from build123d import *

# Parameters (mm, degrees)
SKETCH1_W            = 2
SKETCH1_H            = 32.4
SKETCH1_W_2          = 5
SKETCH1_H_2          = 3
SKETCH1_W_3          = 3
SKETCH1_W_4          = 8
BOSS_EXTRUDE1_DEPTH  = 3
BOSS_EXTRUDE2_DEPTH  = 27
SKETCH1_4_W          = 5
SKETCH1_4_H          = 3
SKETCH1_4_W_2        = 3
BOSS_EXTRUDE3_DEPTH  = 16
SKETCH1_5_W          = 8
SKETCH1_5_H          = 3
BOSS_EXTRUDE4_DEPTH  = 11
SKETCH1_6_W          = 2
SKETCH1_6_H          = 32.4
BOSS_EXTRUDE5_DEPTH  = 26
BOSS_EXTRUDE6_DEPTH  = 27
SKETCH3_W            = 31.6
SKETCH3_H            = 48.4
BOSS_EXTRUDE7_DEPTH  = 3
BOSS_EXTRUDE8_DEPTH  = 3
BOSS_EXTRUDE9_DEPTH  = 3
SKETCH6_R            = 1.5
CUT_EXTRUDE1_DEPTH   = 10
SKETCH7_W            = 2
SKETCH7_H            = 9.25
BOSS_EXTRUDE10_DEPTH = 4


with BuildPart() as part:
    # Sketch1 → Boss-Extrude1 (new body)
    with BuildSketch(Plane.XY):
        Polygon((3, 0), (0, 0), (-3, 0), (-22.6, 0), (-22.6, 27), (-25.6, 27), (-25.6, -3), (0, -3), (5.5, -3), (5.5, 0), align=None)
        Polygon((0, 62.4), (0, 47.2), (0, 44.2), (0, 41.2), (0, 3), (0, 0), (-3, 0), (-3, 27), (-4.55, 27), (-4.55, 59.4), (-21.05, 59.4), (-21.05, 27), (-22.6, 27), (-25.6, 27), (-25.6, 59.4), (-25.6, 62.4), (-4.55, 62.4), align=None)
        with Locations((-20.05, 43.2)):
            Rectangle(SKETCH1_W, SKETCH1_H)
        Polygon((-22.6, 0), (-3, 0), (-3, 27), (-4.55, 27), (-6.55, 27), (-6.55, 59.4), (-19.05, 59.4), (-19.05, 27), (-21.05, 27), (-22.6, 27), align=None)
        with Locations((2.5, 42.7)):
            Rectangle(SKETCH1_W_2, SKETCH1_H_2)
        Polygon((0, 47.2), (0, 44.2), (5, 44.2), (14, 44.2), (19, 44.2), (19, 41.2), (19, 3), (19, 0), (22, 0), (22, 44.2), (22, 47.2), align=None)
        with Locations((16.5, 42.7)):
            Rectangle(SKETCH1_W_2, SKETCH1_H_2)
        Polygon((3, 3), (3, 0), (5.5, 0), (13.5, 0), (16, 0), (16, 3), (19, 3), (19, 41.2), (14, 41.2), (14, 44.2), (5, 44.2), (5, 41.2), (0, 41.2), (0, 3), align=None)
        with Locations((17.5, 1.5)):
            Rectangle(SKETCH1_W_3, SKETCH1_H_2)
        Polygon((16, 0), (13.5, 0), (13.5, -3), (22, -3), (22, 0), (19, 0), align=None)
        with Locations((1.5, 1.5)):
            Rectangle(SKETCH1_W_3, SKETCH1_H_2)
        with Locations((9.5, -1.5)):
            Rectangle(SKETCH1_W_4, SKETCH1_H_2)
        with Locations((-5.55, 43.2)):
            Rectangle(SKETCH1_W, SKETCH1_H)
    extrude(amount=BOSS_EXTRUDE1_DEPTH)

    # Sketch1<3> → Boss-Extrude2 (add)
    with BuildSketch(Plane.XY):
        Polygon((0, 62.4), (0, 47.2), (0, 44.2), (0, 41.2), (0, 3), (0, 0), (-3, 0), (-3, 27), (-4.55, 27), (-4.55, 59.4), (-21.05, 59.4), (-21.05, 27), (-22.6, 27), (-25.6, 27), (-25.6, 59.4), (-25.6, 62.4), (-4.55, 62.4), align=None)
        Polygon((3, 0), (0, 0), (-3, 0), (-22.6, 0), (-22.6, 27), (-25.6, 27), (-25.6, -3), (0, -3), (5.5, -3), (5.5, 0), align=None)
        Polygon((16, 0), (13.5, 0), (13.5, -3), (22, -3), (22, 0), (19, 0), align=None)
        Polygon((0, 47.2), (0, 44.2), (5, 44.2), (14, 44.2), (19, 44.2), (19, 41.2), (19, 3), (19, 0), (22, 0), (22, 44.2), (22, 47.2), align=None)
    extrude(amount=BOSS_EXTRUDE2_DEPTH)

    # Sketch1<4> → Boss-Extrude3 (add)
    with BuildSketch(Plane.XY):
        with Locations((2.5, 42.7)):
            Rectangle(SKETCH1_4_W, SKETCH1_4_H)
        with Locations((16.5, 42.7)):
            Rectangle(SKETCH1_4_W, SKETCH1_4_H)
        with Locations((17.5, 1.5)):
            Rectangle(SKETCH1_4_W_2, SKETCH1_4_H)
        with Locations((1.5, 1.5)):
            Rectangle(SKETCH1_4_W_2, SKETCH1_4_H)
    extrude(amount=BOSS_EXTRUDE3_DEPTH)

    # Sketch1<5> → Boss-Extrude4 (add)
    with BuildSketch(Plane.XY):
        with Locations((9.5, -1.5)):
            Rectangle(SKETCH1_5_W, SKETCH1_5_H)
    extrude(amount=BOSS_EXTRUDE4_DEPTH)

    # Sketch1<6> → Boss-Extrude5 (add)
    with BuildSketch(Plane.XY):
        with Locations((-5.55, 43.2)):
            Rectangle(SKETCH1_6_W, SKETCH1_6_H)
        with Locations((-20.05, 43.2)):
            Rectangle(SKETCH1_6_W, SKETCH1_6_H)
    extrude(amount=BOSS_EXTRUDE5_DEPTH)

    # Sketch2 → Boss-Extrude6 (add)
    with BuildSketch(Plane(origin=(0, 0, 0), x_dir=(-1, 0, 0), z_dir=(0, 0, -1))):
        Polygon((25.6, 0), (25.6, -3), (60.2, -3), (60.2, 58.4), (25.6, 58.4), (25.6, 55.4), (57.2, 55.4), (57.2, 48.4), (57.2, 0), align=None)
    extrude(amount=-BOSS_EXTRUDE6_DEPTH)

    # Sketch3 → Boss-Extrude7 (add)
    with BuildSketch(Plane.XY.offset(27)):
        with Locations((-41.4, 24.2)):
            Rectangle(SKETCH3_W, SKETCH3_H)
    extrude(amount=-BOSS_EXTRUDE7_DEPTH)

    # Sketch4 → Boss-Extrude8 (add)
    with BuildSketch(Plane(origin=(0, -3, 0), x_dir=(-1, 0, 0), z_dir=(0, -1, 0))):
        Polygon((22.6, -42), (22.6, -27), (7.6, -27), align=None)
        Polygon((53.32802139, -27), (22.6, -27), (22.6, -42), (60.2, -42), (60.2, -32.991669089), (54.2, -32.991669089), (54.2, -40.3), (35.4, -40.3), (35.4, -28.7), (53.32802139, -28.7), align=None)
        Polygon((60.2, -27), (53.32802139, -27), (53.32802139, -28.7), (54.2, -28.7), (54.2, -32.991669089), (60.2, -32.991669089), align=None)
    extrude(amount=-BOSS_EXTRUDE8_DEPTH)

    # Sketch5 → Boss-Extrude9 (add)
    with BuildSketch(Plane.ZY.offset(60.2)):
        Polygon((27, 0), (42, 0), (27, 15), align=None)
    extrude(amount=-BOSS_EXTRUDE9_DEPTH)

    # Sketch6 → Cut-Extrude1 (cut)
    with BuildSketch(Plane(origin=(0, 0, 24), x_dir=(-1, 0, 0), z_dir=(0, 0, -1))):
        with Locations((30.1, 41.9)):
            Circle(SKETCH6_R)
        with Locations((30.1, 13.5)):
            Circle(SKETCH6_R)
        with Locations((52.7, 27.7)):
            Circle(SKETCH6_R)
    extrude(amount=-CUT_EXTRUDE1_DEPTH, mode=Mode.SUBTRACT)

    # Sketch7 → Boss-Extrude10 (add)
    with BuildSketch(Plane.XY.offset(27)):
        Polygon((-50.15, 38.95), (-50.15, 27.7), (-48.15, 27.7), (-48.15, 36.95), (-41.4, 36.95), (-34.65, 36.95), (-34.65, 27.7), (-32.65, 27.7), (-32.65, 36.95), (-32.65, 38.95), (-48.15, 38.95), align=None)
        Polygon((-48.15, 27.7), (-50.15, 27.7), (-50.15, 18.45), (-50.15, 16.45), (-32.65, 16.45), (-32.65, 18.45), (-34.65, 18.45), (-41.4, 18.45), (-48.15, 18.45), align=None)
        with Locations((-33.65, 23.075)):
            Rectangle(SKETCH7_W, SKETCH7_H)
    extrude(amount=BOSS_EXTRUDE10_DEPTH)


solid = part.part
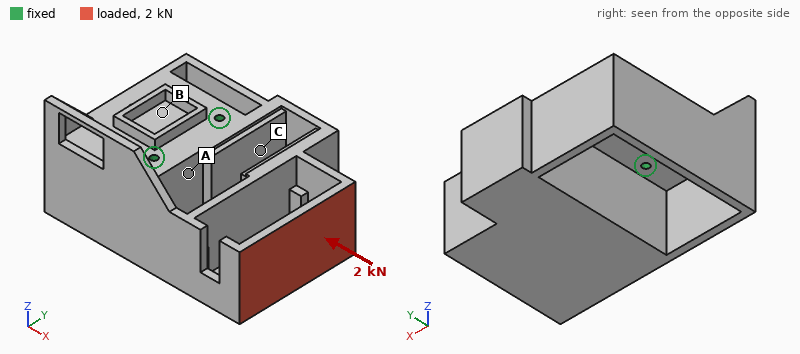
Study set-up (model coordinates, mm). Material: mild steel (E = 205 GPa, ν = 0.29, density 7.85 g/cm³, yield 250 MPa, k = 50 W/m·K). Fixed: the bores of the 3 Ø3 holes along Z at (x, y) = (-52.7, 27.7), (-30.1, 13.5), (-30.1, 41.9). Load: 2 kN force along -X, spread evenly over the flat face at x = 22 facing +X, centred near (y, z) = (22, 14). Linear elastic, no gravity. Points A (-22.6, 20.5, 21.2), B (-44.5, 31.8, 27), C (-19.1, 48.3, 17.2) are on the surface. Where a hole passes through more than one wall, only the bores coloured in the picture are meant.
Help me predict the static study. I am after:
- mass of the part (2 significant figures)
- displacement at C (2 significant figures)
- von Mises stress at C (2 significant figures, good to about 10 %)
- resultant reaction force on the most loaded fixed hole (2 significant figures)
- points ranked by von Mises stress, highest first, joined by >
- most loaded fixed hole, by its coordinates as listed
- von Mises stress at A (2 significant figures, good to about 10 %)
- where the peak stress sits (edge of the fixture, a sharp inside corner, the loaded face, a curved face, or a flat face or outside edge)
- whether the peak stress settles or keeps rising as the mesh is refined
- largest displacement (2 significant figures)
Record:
390 g
14 µm
32 MPa
1.1 kN
C > A > B
(-30.1, 13.5)
15 MPa
edge of the fixture
keeps rising
88 µm
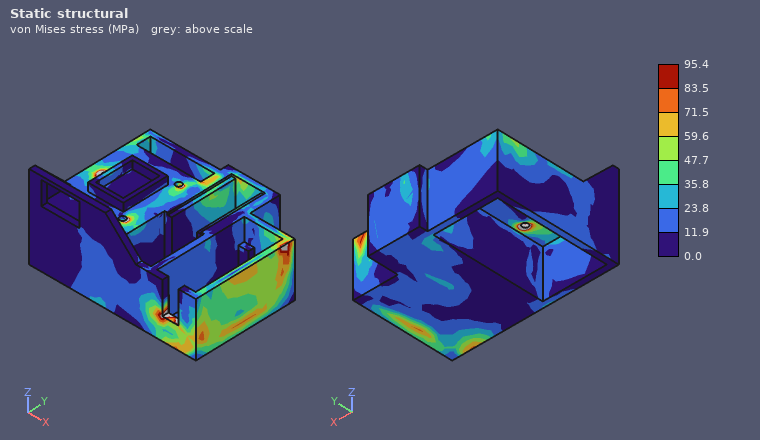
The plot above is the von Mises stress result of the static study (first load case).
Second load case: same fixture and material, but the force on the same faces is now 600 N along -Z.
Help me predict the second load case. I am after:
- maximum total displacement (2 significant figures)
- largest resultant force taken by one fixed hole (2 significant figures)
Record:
69 µm
1.0 kN
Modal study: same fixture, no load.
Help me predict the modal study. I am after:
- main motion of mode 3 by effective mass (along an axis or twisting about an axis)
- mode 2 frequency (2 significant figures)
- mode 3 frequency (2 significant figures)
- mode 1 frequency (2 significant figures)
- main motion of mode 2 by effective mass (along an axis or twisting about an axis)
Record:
along Y
1800 Hz
2700 Hz
1600 Hz
along Y
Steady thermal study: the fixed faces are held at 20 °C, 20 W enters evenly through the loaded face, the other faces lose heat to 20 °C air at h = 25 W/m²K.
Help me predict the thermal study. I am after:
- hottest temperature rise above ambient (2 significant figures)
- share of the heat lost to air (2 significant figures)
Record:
70 K
66 %
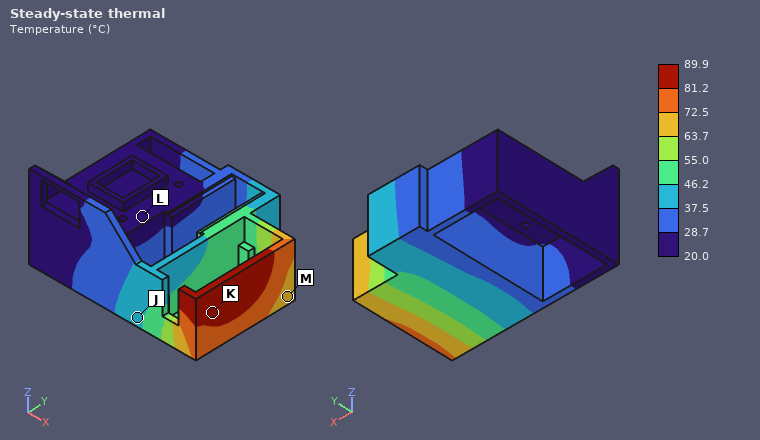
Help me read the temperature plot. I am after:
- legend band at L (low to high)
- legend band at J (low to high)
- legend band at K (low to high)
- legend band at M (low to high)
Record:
20.0 to 28.7 °C
37.5 to 46.2 °C
81.2 to 89.9 °C
63.7 to 72.5 °C
